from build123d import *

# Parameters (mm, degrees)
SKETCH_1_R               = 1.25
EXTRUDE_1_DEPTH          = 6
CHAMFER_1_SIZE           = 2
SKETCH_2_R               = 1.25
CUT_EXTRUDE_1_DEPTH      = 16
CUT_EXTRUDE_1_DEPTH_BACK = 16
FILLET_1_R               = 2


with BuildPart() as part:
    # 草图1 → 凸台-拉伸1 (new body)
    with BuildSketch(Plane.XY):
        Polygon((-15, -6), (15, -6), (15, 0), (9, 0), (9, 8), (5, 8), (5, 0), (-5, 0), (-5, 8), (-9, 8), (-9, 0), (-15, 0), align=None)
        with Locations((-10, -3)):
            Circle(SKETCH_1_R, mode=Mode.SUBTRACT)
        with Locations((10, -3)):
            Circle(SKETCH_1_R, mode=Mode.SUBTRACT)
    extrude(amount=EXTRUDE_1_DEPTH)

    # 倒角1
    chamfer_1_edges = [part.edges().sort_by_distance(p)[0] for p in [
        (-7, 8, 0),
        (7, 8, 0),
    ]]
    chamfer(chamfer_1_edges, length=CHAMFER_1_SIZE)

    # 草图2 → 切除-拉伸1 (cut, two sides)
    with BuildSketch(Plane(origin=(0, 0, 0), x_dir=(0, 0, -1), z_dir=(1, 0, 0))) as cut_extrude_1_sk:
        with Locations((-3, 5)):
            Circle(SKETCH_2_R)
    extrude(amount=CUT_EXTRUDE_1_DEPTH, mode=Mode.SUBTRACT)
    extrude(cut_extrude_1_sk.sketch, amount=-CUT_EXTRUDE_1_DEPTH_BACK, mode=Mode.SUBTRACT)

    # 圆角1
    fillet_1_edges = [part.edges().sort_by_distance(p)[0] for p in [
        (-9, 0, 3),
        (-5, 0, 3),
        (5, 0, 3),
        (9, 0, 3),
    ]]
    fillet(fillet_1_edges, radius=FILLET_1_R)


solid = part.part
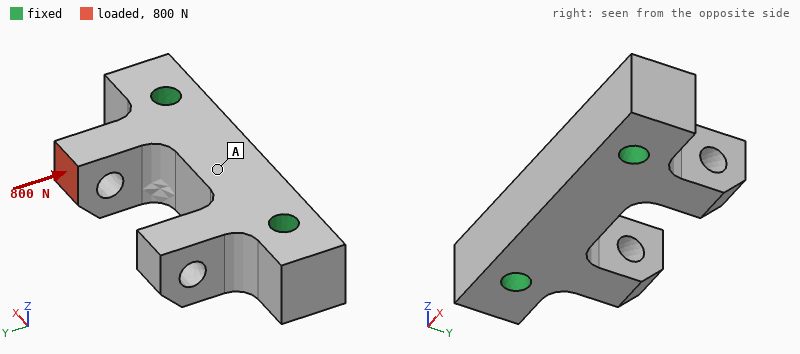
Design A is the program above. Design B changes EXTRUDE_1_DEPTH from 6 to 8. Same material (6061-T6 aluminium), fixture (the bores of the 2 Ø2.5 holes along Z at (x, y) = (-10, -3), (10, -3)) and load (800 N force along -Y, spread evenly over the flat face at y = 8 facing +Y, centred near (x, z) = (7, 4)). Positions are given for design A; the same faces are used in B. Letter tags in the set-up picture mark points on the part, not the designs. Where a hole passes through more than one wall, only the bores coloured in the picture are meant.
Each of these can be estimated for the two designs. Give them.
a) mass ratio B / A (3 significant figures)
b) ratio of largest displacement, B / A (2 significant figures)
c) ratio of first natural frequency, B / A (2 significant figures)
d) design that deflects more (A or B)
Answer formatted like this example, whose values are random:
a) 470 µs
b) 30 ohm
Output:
a) 1.35
b) 0.60
c) 0.98
d) A
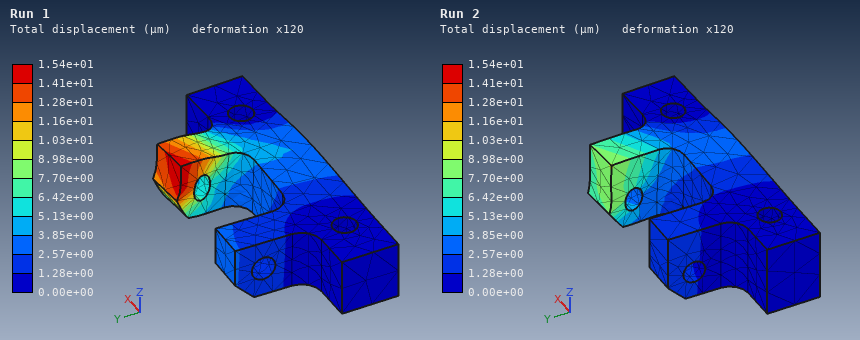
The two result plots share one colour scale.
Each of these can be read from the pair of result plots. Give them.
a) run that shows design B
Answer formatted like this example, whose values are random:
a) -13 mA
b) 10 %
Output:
a) Run 2
